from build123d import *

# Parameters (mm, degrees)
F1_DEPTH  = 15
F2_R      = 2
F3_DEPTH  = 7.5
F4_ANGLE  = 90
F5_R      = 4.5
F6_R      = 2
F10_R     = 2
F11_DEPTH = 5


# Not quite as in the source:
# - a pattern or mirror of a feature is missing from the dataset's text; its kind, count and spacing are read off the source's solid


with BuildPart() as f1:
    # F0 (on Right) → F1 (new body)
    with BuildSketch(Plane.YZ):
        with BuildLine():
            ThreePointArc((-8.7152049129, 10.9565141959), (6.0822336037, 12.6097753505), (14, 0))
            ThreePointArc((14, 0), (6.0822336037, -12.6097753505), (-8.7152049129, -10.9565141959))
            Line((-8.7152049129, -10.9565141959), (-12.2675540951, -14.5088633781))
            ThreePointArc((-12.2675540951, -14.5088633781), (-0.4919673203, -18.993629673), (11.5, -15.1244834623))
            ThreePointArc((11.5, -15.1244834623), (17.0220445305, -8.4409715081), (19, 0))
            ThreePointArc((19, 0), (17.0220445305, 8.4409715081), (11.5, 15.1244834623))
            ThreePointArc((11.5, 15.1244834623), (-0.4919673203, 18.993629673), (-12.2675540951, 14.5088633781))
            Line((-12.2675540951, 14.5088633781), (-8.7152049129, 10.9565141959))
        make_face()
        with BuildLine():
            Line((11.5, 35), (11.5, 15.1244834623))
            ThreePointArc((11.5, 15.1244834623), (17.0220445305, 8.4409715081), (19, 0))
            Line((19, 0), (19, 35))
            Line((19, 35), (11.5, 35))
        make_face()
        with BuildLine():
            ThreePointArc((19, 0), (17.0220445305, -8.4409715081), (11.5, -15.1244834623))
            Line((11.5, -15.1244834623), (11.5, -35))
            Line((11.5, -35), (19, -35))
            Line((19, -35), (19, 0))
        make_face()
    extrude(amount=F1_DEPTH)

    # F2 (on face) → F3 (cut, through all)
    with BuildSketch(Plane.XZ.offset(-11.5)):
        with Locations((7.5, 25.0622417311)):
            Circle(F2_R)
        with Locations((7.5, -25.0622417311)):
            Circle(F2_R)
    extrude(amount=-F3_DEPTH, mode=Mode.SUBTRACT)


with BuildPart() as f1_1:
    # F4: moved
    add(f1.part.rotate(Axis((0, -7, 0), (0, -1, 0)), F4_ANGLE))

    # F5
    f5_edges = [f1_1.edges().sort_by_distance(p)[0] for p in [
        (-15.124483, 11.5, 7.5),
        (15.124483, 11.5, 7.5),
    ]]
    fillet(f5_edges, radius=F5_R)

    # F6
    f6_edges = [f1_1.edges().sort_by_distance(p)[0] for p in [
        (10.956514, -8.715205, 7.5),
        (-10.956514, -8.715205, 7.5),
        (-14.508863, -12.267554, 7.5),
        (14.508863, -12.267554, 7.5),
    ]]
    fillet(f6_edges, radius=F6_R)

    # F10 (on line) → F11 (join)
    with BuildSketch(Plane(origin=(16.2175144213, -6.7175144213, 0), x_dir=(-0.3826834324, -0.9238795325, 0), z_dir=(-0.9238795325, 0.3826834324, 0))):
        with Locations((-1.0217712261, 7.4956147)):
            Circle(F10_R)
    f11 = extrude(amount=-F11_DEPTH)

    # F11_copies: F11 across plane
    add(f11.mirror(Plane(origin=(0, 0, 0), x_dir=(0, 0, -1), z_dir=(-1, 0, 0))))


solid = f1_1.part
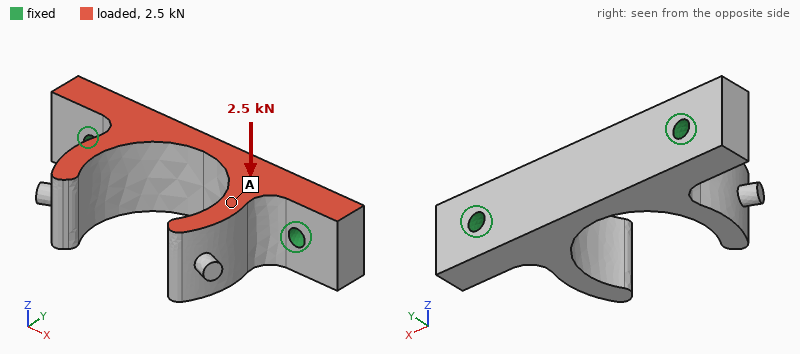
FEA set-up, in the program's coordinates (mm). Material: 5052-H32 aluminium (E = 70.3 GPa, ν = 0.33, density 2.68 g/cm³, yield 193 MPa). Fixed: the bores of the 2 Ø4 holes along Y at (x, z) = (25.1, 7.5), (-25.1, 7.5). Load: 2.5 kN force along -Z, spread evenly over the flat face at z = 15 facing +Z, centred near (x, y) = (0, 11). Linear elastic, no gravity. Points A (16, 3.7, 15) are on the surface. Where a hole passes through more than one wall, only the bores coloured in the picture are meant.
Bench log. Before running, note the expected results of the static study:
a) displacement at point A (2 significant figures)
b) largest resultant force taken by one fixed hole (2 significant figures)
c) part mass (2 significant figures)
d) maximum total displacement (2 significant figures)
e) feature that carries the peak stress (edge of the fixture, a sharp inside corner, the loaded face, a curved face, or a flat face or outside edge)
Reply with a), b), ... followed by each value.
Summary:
a) 22 µm
b) 1.3 kN
c) 30 g
d) 42 µm
e) edge of the fixture
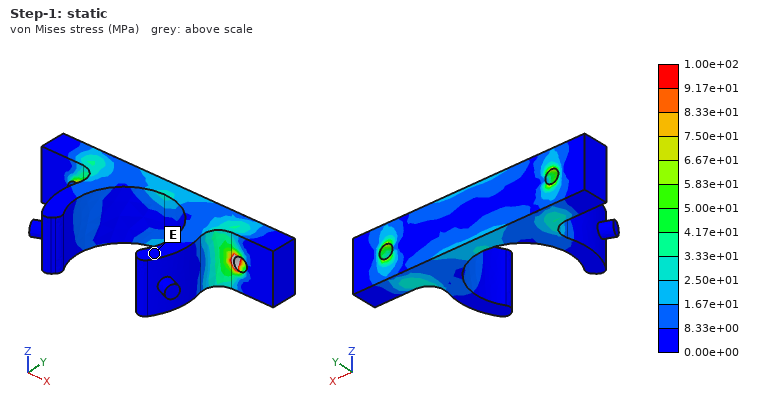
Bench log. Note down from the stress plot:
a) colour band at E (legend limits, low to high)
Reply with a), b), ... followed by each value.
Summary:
a) 0.00e+00 to 8.33e+00 MPa
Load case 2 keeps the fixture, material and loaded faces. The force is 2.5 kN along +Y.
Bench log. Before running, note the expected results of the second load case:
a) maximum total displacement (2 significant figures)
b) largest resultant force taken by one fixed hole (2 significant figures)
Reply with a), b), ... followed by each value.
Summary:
a) 57 µm
b) 1.3 kN
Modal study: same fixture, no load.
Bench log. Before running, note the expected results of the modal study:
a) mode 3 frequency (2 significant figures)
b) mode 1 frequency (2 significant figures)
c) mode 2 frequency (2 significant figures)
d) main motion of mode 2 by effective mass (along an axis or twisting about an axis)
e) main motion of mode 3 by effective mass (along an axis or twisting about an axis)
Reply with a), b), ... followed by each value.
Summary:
a) 9100 Hz
b) 6900 Hz
c) 8500 Hz
d) along Z
e) along X
